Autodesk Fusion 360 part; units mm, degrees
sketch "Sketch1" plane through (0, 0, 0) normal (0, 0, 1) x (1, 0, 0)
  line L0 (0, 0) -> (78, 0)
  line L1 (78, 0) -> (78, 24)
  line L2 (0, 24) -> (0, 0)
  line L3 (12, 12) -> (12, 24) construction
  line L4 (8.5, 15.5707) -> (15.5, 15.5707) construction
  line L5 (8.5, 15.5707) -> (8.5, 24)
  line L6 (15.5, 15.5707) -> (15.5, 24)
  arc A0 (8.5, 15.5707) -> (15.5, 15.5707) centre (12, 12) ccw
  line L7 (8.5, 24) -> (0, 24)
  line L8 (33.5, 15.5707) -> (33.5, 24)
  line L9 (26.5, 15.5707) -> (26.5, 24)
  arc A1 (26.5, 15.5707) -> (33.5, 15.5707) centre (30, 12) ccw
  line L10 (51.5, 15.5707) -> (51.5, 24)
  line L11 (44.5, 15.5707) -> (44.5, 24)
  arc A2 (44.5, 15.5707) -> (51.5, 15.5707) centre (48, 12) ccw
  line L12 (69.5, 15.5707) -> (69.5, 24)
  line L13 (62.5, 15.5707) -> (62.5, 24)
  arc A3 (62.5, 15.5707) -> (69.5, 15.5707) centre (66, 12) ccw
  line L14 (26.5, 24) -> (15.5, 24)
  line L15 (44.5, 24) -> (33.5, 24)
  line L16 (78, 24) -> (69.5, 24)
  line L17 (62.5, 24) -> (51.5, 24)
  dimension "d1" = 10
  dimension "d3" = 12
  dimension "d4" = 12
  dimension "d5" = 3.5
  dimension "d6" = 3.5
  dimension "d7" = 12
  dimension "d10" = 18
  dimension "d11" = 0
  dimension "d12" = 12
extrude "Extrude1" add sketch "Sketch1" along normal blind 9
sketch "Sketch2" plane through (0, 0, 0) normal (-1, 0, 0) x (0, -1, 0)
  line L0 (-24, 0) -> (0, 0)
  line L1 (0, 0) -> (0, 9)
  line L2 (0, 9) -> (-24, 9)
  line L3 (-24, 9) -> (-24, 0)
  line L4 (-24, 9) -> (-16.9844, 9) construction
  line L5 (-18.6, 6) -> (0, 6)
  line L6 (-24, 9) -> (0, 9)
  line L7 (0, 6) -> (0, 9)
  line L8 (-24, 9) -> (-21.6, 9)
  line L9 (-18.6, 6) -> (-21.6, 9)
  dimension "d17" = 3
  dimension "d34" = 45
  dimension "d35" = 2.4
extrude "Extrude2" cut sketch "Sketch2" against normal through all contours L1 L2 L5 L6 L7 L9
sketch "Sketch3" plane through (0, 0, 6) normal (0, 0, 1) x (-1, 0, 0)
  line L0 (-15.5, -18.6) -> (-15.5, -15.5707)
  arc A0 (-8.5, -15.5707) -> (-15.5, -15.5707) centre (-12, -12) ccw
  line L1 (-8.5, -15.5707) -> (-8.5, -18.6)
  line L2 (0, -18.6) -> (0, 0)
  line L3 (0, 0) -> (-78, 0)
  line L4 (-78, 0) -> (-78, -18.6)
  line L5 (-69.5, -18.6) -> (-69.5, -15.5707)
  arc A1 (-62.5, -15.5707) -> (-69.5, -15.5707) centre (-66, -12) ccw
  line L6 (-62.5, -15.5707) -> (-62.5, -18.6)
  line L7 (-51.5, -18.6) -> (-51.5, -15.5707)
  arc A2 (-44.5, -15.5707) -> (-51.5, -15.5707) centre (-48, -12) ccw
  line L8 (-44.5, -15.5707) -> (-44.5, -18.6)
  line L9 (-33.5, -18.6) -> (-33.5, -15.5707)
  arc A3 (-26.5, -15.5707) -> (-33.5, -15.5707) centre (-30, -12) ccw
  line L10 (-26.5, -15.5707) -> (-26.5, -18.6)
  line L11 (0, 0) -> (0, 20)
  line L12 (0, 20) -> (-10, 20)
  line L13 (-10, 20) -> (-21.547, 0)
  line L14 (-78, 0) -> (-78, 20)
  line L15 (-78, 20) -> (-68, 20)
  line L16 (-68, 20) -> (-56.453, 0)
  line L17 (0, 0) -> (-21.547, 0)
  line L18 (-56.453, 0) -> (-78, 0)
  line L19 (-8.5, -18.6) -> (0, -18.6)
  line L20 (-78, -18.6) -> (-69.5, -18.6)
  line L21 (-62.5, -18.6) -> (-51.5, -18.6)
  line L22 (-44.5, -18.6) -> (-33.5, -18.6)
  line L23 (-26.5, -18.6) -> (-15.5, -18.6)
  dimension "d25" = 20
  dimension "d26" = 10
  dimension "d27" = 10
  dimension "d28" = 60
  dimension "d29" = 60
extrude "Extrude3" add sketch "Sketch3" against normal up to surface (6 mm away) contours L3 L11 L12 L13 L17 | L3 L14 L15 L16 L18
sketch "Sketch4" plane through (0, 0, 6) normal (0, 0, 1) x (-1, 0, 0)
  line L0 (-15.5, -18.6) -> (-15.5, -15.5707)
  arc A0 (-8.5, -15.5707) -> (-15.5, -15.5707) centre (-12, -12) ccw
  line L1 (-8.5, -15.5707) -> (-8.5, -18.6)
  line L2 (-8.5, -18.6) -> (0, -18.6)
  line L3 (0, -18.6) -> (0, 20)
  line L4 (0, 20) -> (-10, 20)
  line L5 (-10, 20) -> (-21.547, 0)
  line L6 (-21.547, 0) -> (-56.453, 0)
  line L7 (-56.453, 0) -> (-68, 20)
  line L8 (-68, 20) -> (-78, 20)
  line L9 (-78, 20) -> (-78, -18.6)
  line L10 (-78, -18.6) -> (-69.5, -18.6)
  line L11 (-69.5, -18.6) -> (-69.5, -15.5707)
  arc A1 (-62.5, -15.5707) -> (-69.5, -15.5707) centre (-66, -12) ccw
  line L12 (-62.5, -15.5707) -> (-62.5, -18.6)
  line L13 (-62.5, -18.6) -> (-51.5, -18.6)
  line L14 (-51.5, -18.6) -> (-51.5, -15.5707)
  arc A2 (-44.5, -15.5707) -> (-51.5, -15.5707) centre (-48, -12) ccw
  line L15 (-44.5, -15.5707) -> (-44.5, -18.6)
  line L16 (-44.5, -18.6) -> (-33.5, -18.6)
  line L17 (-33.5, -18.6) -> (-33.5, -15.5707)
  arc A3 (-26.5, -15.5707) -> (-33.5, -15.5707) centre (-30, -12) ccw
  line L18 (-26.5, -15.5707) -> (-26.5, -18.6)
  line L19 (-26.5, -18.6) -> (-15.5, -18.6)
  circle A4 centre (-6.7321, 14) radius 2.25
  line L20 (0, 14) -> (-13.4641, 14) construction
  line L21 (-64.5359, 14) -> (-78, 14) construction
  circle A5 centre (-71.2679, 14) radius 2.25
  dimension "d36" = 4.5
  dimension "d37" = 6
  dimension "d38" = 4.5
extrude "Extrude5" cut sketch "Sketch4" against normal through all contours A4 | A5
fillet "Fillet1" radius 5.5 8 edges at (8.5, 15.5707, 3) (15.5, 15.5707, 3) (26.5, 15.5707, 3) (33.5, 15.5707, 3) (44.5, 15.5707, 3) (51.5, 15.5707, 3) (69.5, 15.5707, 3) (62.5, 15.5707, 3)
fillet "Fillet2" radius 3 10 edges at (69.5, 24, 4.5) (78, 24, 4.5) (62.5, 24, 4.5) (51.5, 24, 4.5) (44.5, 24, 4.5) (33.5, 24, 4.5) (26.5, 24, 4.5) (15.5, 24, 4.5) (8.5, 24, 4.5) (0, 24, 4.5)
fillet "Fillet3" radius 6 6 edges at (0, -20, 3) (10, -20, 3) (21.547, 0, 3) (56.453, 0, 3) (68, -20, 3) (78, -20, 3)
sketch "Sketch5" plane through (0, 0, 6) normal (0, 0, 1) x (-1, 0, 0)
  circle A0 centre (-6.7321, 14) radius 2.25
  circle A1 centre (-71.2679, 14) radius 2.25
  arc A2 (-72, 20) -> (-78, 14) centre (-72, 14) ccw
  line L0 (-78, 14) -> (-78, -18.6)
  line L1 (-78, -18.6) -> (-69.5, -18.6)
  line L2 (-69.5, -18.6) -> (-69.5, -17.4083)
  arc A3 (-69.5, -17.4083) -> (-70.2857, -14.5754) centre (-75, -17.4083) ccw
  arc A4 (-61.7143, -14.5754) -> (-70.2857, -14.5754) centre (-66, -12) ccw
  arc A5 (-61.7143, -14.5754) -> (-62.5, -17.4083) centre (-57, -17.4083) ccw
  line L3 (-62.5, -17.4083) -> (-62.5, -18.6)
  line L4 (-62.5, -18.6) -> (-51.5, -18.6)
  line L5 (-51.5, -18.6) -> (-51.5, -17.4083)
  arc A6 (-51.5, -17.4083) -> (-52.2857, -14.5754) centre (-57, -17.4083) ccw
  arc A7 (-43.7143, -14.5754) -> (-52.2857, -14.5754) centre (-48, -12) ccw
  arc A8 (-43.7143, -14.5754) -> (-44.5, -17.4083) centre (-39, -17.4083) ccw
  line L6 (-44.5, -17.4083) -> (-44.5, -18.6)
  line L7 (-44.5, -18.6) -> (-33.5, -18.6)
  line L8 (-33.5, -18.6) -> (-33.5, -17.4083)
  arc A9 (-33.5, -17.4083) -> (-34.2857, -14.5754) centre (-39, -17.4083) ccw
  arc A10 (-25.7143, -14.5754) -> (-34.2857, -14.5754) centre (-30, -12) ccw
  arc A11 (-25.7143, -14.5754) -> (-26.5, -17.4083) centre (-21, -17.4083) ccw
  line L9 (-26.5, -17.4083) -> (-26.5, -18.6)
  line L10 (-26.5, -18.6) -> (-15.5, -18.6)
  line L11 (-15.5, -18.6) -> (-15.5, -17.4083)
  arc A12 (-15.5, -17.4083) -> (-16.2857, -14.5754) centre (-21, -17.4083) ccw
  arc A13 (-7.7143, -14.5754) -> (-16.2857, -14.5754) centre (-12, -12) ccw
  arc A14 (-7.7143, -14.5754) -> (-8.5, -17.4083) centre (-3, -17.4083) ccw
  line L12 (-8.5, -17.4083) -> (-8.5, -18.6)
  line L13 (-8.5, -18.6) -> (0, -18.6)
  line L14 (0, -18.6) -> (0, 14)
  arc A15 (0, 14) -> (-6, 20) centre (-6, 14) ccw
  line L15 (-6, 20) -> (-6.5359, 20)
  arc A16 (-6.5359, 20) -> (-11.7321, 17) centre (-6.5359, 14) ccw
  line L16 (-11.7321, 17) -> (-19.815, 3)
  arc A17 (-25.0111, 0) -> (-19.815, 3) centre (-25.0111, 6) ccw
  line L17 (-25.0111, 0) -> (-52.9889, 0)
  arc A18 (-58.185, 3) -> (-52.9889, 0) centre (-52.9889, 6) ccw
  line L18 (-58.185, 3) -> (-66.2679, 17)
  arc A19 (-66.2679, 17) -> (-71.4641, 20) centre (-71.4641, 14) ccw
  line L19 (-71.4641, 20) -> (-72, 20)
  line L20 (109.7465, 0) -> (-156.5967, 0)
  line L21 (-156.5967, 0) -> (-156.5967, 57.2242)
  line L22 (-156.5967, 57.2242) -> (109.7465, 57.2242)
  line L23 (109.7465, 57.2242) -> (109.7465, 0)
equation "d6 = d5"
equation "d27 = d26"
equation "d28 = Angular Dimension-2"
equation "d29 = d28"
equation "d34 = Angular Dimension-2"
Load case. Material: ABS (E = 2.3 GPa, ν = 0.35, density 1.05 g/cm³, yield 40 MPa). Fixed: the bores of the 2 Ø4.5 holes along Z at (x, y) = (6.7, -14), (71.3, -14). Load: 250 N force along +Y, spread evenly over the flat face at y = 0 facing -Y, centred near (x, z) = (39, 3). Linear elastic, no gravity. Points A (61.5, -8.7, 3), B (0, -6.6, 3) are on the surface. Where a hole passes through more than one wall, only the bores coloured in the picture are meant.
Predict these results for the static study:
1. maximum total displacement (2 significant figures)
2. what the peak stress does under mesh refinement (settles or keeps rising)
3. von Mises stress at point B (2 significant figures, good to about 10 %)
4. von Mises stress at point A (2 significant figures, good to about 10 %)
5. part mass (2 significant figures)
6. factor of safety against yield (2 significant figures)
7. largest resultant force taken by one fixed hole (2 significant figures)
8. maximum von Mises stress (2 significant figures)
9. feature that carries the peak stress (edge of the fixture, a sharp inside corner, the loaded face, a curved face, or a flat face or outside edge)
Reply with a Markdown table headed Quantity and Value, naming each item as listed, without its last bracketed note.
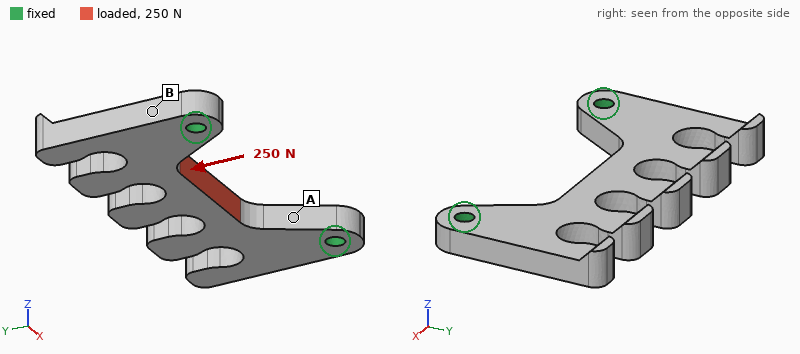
| Quantity | Value |
|---|---|
| maximum total displacement | 0.20 mm |
| what the peak stress does under mesh refinement | settles |
| von Mises stress at point B | 1.9 MPa |
| von Mises stress at point A | 5.4 MPa |
| part mass | 13 g |
| factor of safety against yield | 2.4 |
| largest resultant force taken by one fixed hole | 180 N |
| maximum von Mises stress | 17 MPa |
| feature that carries the peak stress | a curved face |
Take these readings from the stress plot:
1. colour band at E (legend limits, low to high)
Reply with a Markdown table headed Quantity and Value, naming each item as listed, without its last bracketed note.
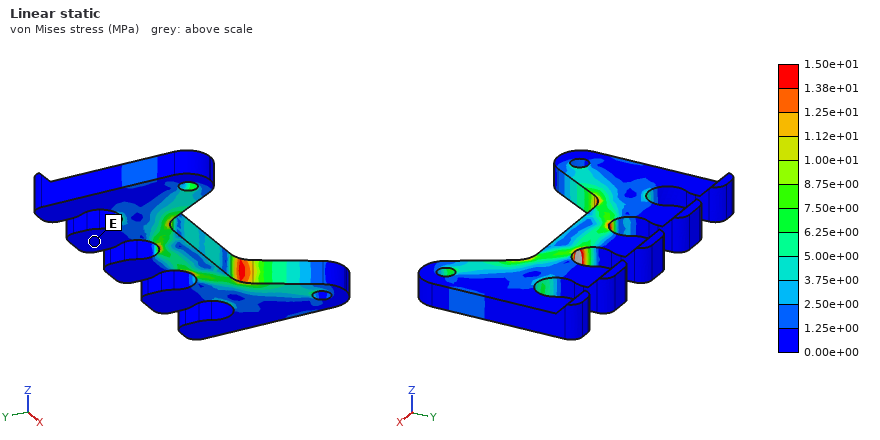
| Quantity | Value |
|---|---|
| colour band at E | 0.00e+00 to 1.25e+00 MPa |
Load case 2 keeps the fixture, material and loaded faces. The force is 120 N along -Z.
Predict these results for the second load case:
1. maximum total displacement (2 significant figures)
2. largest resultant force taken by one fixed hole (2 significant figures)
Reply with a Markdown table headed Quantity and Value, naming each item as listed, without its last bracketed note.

| Quantity | Value |
|---|---|
| maximum total displacement | 0.65 mm |
| largest resultant force taken by one fixed hole | 60 N |
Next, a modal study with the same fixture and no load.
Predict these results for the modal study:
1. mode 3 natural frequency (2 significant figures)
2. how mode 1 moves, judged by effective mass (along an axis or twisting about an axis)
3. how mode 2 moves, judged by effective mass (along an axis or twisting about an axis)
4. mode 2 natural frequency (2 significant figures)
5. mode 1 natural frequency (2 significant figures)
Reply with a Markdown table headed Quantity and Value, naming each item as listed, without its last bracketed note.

| Quantity | Value |
|---|---|
| mode 3 natural frequency | 1400 Hz |
| how mode 1 moves, judged by effective mass | along Z |
| how mode 2 moves, judged by effective mass | twisting about Y |
| mode 2 natural frequency | 1100 Hz |
| mode 1 natural frequency | 680 Hz |
